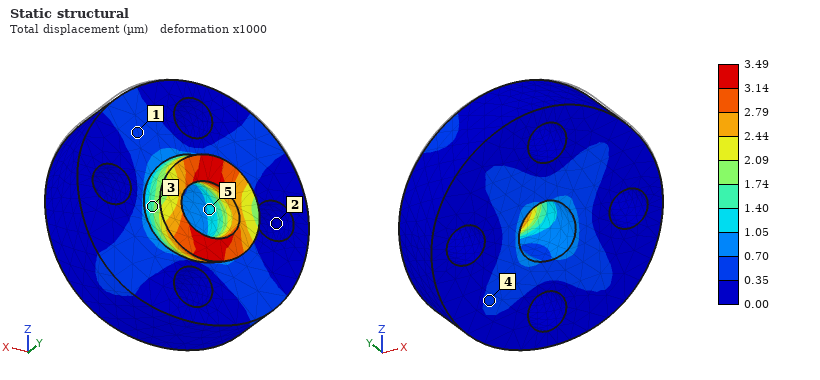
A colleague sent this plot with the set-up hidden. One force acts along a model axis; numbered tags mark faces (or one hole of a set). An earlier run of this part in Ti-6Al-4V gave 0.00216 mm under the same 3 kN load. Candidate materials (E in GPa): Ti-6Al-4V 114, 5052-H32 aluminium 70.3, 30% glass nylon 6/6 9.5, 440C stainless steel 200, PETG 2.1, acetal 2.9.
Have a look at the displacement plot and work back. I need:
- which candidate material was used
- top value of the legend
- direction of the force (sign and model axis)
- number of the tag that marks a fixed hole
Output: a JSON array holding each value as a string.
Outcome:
["5052-H32 aluminium", "3.49 µm", "-Z", "2"]
